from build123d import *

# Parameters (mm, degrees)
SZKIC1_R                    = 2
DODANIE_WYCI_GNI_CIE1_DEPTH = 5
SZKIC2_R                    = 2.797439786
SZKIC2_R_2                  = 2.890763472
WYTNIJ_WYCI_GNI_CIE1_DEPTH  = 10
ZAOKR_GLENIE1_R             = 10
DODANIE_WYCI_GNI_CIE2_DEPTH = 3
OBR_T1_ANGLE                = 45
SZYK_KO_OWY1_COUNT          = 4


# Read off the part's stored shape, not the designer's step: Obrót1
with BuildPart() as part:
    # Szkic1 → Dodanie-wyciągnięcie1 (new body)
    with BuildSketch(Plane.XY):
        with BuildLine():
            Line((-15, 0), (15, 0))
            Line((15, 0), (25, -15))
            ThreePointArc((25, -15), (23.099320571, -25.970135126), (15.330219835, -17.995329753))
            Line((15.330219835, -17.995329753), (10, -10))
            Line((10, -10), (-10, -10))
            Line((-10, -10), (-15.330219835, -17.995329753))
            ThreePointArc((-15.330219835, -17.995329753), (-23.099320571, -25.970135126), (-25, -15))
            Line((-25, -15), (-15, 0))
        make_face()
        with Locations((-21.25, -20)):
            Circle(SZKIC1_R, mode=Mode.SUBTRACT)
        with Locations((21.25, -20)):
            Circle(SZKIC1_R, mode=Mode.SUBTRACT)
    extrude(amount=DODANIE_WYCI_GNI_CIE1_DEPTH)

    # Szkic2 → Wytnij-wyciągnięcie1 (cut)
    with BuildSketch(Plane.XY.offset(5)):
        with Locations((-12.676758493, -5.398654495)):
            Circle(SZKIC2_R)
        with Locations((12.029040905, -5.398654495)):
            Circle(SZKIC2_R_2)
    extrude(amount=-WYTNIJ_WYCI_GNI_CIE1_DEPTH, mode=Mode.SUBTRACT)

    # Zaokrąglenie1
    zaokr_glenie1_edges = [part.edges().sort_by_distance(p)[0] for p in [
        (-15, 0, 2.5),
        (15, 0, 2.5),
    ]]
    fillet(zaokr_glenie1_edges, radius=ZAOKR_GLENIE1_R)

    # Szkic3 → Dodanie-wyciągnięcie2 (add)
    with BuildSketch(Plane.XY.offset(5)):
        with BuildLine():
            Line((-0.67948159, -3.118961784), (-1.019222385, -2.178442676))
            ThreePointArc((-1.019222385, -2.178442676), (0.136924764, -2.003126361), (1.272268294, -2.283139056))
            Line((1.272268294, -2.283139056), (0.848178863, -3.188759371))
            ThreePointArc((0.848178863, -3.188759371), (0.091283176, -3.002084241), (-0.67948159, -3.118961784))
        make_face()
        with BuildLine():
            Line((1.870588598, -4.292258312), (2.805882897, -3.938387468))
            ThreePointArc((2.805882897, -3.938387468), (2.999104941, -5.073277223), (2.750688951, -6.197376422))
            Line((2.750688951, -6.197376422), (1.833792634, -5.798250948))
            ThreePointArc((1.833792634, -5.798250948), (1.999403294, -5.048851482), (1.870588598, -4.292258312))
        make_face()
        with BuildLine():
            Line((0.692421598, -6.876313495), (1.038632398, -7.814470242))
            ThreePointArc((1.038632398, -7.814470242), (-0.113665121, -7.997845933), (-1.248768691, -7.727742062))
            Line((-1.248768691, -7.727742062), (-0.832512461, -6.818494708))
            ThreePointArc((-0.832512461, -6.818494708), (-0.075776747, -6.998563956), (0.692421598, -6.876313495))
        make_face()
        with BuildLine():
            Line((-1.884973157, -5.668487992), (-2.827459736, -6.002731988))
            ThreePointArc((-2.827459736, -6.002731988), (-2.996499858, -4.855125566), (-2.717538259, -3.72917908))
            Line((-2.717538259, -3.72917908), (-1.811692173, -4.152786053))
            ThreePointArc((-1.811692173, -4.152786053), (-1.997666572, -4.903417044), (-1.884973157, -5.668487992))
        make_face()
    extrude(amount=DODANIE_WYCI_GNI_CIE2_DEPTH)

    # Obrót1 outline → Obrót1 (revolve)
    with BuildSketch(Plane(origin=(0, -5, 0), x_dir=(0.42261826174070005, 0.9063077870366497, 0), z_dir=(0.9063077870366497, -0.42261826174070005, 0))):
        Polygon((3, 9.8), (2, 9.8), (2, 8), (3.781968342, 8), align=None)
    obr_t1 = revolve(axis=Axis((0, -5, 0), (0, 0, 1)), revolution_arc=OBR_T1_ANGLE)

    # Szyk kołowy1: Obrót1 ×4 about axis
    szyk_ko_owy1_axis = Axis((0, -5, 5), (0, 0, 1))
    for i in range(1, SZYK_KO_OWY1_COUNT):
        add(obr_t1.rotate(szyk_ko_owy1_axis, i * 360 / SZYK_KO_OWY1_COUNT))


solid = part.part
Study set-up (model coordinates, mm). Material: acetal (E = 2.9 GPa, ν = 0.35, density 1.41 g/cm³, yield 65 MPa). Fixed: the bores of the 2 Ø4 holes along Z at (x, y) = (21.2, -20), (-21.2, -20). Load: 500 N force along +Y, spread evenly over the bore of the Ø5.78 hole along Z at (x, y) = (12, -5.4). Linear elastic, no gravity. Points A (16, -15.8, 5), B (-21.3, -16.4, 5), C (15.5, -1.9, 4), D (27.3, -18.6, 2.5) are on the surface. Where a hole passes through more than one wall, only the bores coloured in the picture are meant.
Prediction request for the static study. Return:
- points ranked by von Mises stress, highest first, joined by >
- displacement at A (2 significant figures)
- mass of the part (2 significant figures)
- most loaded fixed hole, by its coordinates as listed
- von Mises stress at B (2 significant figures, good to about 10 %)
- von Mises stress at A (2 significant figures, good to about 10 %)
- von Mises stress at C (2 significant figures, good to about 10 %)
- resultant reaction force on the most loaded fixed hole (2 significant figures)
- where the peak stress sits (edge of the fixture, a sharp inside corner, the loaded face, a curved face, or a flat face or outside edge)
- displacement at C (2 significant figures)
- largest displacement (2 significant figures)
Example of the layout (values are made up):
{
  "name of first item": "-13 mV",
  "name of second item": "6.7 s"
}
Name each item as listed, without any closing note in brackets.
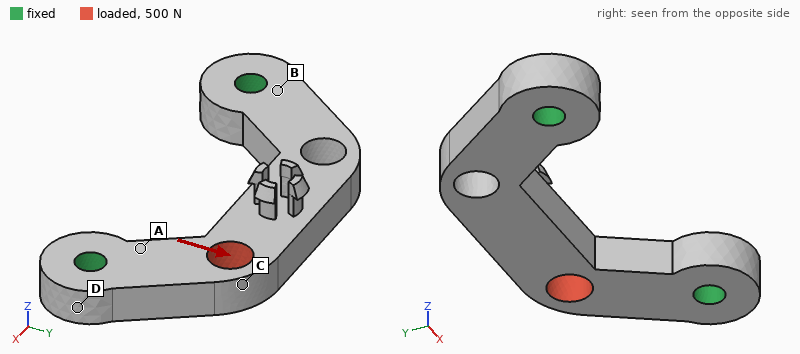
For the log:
{
  "points ranked by von Mises stress, highest first, joined by >": "A > C > B > D",
  "displacement at A": "0.044 mm",
  "mass of the part": "4.6 g",
  "most loaded fixed hole, by its coordinates as listed": "(21.2, -20)",
  "von Mises stress at B": "5.0 MPa",
  "von Mises stress at A": "12 MPa",
  "von Mises stress at C": "8.9 MPa",
  "resultant reaction force on the most loaded fixed hole": "450 N",
  "where the peak stress sits": "the loaded face",
  "displacement at C": "0.10 mm",
  "largest displacement": "0.16 mm"
}
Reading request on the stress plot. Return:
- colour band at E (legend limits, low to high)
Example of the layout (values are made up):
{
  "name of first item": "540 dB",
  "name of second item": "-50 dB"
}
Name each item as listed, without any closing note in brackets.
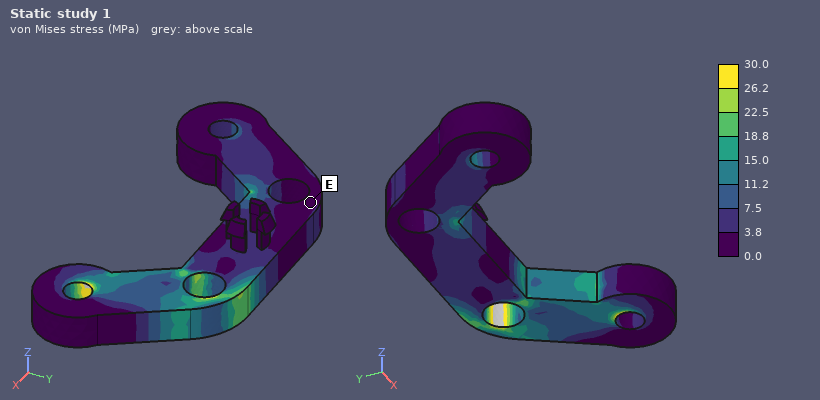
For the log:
{
  "colour band at E": "0.0 to 3.8 MPa"
}
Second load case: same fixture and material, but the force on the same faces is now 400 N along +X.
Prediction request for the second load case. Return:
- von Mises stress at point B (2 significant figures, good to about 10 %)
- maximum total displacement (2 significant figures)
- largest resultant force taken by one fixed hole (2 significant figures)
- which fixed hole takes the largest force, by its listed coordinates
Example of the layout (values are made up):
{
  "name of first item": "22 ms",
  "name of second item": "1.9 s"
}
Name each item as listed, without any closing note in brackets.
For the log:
{
  "von Mises stress at point B": "7.7 MPa",
  "maximum total displacement": "0.15 mm",
  "largest resultant force taken by one fixed hole": "240 N",
  "which fixed hole takes the largest force, by its listed coordinates": "(21.2, -20)"
}
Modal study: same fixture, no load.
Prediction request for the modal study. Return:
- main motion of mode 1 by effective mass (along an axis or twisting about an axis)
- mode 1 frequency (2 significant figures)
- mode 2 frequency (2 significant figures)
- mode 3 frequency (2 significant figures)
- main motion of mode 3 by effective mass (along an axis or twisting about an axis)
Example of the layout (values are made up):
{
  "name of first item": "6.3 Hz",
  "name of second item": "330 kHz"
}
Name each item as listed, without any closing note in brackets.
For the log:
{
  "main motion of mode 1 by effective mass": "along Z",
  "mode 1 frequency": "1900 Hz",
  "mode 2 frequency": "4600 Hz",
  "mode 3 frequency": "6000 Hz",
  "main motion of mode 3 by effective mass": "along X"
}
